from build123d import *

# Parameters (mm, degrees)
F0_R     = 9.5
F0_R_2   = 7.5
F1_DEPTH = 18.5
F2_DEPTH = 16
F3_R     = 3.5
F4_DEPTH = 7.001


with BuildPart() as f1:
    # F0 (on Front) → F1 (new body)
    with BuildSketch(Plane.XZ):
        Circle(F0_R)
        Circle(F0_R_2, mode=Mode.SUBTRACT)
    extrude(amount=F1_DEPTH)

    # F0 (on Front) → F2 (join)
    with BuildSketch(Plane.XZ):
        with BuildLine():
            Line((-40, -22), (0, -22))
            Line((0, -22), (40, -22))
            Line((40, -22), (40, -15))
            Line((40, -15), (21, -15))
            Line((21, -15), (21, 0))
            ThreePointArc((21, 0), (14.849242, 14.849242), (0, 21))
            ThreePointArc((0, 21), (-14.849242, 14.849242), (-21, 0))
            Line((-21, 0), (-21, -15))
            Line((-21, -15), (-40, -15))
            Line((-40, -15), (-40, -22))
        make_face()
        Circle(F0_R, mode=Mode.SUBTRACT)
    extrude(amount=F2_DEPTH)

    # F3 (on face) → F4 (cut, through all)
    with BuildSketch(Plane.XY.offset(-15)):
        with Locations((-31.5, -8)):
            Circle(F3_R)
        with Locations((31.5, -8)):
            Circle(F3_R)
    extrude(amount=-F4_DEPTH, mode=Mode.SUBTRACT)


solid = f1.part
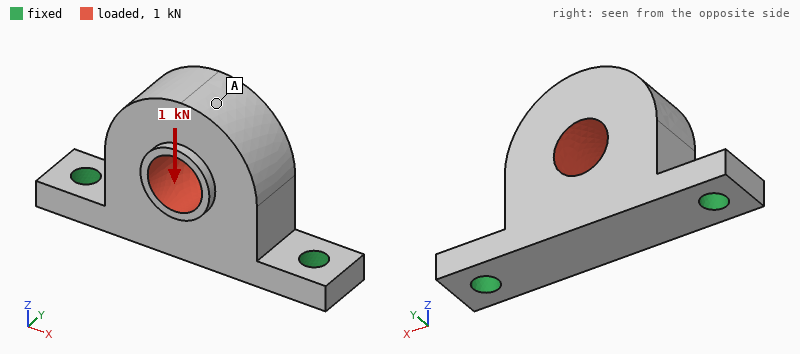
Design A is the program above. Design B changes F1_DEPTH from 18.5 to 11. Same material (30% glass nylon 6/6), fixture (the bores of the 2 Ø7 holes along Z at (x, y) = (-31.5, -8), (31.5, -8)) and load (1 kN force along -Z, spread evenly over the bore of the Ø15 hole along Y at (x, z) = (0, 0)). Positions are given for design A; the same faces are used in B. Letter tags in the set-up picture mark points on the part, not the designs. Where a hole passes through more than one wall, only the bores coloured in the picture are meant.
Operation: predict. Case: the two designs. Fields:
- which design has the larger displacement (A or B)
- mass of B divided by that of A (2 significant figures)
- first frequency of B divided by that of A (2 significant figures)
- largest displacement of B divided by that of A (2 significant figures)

B
0.97
1.0
1.7
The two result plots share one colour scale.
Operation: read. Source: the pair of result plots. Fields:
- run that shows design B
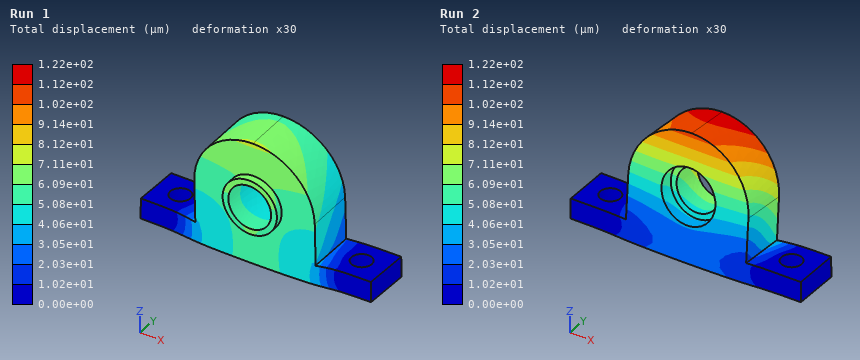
Run 2
